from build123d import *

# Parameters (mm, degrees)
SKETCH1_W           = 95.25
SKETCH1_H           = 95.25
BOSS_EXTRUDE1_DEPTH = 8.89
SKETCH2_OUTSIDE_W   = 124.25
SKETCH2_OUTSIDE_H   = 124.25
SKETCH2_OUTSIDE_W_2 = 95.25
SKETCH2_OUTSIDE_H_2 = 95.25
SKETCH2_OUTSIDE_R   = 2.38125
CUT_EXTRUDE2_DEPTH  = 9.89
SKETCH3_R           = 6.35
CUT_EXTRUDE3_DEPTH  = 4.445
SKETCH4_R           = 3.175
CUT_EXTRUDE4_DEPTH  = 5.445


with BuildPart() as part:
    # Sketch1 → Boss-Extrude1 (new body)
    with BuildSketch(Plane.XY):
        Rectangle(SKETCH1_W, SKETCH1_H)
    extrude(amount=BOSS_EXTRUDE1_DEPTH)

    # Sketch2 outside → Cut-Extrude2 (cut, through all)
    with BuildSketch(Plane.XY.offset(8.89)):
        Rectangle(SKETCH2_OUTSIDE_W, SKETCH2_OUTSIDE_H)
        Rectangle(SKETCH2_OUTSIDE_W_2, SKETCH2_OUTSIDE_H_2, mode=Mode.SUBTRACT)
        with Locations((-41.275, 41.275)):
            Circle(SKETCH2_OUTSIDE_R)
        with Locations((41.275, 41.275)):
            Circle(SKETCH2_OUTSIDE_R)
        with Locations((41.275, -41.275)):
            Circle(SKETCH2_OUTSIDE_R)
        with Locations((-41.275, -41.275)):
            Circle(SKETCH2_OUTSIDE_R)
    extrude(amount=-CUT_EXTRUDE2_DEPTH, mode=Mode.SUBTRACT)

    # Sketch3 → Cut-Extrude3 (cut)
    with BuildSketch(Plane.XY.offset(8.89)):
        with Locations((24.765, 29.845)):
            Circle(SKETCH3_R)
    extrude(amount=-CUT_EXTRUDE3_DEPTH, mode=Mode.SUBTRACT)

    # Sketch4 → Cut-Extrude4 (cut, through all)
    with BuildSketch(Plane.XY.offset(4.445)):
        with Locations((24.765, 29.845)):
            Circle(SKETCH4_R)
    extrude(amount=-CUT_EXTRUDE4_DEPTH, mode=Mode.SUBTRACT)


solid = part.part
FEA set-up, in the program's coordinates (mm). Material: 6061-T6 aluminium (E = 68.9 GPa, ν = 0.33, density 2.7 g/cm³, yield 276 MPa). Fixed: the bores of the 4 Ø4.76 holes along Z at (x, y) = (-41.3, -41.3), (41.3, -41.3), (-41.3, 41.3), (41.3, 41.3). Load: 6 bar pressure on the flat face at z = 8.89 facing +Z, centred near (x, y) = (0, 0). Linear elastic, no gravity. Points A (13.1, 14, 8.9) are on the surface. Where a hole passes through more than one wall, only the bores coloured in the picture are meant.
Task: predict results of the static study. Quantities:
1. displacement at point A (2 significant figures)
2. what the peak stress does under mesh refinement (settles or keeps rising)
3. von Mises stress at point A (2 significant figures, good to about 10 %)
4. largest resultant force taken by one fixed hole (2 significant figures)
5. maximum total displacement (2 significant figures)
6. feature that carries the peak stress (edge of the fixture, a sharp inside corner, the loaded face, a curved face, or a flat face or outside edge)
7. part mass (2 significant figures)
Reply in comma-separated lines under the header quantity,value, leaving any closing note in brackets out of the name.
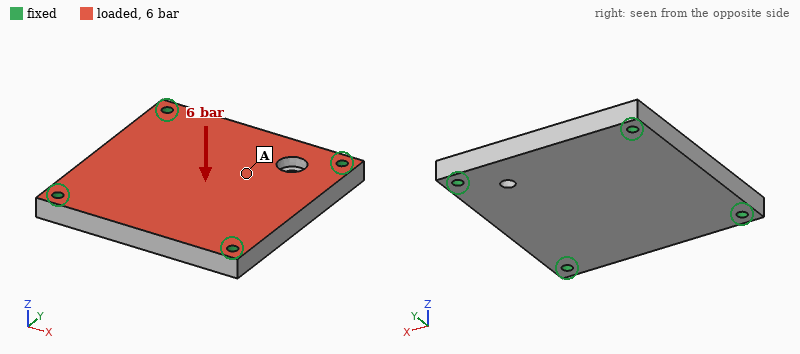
quantity,value
displacement at point A,51 µm
what the peak stress does under mesh refinement,keeps rising
von Mises stress at point A,15 MPa
largest resultant force taken by one fixed hole,1.3 kN
maximum total displacement,58 µm
feature that carries the peak stress,edge of the fixture
part mass,210 g
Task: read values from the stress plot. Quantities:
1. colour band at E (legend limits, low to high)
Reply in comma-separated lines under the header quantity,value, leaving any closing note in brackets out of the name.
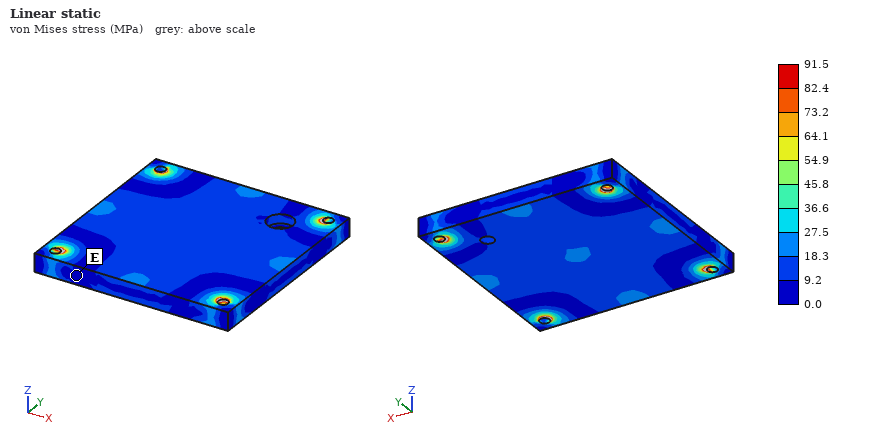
quantity,value
colour band at E,0.0 to 9.2 MPa
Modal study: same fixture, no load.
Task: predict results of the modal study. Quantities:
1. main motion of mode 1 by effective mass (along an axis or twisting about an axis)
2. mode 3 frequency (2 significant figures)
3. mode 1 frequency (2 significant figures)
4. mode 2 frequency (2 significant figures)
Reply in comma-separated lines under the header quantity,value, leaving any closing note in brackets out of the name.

quantity,value
main motion of mode 1 by effective mass,along Z
mode 3 frequency,6700 Hz
mode 1 frequency,3900 Hz
mode 2 frequency,6700 Hz
